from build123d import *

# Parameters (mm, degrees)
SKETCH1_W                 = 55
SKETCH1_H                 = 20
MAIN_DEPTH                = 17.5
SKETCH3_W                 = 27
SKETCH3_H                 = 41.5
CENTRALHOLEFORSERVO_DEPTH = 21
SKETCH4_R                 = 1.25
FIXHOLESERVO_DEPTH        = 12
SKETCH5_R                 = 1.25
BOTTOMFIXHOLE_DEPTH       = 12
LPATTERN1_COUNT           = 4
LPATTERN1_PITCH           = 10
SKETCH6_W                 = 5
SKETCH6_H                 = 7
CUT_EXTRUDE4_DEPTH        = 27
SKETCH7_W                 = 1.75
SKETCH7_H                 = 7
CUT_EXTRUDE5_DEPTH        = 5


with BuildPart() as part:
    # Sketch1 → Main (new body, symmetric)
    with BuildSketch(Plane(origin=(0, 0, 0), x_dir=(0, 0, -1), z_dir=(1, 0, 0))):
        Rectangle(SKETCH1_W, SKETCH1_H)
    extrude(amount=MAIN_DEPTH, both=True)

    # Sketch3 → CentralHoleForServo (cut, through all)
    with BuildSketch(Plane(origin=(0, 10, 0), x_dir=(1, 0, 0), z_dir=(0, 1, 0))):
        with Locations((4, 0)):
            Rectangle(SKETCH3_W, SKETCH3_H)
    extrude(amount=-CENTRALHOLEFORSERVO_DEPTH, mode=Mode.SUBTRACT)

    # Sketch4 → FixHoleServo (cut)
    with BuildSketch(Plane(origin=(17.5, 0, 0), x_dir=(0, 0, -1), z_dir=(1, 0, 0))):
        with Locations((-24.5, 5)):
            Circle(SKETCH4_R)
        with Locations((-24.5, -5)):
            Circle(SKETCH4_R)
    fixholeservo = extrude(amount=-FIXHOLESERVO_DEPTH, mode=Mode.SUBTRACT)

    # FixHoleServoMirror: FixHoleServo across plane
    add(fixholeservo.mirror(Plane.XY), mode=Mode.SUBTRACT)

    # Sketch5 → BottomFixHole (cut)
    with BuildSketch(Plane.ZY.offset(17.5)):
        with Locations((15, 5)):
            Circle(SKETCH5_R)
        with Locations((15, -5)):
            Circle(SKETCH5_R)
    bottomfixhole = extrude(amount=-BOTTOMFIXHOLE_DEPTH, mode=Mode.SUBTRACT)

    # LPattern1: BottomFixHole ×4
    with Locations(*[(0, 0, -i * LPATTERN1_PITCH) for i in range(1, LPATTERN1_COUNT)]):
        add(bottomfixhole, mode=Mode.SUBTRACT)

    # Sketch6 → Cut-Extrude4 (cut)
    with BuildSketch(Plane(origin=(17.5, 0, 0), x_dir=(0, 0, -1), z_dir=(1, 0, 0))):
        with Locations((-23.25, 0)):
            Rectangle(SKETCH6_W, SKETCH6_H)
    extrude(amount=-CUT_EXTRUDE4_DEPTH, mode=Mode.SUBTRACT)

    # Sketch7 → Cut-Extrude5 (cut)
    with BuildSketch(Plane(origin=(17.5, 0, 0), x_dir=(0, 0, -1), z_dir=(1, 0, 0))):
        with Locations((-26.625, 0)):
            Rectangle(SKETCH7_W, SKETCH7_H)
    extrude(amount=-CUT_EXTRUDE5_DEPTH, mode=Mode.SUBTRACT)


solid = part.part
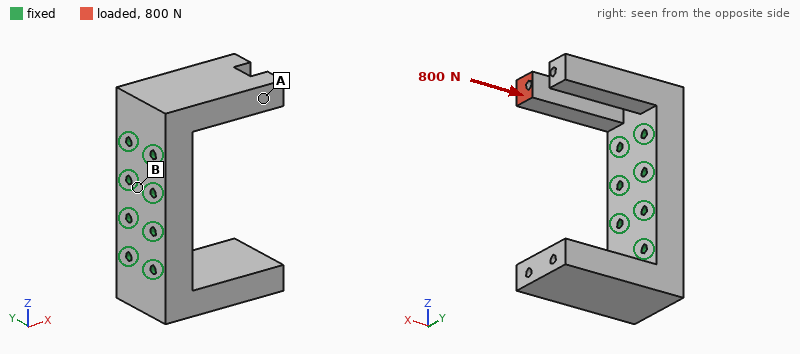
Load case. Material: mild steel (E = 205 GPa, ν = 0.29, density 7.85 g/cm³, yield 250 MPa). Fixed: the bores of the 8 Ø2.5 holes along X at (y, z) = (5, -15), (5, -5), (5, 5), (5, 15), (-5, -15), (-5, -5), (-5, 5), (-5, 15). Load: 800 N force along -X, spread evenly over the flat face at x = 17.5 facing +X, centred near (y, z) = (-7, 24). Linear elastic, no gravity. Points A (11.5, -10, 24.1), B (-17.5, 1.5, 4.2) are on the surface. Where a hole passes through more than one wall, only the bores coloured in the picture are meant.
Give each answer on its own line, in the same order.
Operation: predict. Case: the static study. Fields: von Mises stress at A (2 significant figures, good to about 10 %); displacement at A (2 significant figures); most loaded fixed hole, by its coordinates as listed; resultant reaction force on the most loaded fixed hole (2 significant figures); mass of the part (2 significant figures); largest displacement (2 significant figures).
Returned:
21 MPa
10 µm
(-5, 15)
790 N
110 g
12 µm
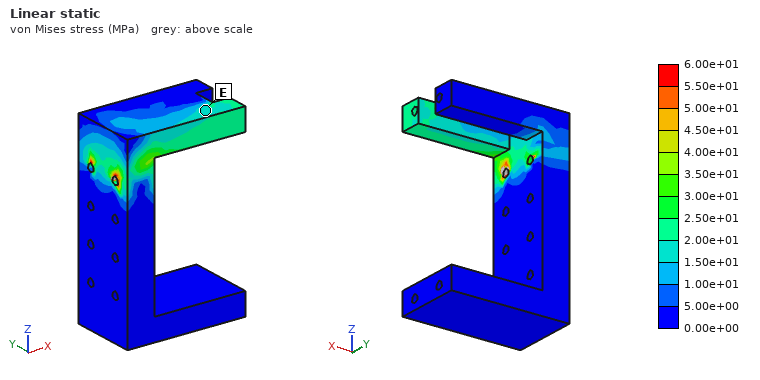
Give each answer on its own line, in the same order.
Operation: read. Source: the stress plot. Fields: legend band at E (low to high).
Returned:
1.50e+01 to 2.00e+01 MPa
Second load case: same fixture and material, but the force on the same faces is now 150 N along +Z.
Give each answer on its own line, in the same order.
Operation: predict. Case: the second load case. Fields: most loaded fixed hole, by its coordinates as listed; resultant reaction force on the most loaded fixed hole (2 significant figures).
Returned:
(-5, 15)
140 N
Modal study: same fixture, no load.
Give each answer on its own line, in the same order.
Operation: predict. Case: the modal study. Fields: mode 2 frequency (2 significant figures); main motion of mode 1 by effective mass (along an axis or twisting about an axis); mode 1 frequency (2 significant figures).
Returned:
5400 Hz
along Z
4800 Hz
